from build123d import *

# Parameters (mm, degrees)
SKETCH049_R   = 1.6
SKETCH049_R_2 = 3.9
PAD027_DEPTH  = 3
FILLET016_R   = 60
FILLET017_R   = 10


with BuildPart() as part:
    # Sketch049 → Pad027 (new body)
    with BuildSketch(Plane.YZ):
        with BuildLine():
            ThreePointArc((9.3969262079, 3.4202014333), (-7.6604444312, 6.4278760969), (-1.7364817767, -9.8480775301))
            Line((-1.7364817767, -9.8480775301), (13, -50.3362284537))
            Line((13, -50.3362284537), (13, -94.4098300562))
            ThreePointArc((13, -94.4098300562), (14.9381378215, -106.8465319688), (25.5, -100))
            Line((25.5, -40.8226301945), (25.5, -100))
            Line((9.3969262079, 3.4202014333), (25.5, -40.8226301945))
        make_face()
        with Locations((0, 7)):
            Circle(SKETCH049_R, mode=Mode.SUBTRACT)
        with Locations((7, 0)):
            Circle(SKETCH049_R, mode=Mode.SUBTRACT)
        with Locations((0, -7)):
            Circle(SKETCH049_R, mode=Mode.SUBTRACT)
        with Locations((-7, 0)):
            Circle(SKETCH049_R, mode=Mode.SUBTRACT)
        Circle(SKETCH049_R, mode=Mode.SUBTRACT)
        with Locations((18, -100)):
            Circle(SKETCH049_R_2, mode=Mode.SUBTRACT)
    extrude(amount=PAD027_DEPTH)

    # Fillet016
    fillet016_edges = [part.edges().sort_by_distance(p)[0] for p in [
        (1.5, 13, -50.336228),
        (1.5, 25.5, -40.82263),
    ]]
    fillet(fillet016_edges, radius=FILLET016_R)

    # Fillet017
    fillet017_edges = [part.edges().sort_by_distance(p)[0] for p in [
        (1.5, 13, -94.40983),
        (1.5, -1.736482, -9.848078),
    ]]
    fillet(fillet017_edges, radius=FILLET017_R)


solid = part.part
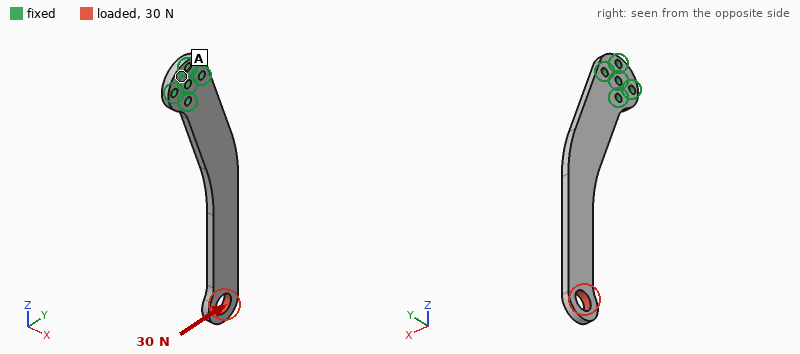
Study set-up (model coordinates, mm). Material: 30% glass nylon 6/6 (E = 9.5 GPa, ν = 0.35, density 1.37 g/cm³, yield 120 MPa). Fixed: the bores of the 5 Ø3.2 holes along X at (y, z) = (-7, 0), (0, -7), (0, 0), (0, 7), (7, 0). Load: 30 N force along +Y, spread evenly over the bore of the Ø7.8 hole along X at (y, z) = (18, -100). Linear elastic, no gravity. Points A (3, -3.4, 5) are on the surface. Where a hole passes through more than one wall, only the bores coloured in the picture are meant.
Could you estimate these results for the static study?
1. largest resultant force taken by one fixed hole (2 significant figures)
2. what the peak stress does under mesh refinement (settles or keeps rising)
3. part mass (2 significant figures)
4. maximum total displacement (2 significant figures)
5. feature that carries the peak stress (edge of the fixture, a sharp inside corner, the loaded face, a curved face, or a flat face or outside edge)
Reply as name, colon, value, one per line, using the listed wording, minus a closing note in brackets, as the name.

largest resultant force taken by one fixed hole: 240 N
what the peak stress does under mesh refinement: keeps rising
part mass: 6.7 g
maximum total displacement: 1.4 mm
feature that carries the peak stress: edge of the fixture
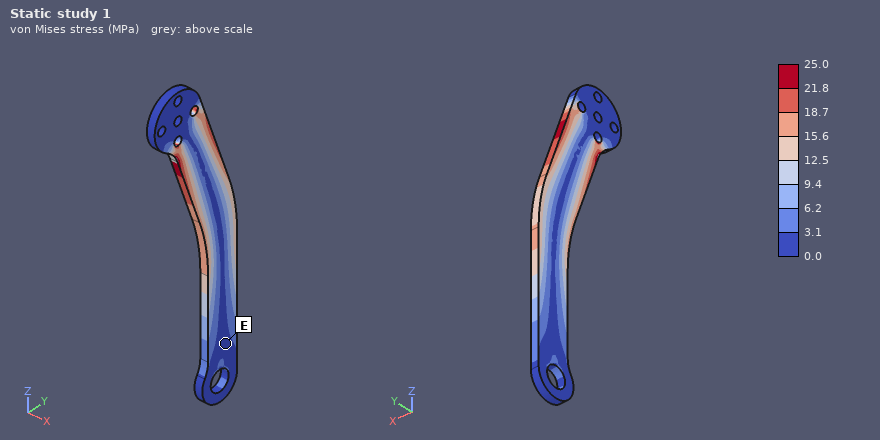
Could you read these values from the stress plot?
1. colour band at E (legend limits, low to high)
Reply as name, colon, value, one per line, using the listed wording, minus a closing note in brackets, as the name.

colour band at E: 0.0 to 3.1 MPa
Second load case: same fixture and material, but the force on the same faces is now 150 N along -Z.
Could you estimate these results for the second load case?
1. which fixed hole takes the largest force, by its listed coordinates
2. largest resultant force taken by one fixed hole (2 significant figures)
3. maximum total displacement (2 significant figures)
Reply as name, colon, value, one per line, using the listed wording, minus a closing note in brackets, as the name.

which fixed hole takes the largest force, by its listed coordinates: (7, 0)
largest resultant force taken by one fixed hole: 230 N
maximum total displacement: 0.44 mm
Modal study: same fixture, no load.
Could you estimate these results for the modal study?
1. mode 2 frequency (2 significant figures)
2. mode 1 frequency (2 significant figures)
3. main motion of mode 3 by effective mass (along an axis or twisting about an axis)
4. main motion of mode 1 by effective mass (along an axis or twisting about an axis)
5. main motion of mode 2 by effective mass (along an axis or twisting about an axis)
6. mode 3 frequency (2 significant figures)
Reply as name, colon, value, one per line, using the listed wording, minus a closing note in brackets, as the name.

mode 2 frequency: 650 Hz
mode 1 frequency: 140 Hz
main motion of mode 3 by effective mass: along X
main motion of mode 1 by effective mass: along X
main motion of mode 2 by effective mass: along Y
mode 3 frequency: 730 Hz
